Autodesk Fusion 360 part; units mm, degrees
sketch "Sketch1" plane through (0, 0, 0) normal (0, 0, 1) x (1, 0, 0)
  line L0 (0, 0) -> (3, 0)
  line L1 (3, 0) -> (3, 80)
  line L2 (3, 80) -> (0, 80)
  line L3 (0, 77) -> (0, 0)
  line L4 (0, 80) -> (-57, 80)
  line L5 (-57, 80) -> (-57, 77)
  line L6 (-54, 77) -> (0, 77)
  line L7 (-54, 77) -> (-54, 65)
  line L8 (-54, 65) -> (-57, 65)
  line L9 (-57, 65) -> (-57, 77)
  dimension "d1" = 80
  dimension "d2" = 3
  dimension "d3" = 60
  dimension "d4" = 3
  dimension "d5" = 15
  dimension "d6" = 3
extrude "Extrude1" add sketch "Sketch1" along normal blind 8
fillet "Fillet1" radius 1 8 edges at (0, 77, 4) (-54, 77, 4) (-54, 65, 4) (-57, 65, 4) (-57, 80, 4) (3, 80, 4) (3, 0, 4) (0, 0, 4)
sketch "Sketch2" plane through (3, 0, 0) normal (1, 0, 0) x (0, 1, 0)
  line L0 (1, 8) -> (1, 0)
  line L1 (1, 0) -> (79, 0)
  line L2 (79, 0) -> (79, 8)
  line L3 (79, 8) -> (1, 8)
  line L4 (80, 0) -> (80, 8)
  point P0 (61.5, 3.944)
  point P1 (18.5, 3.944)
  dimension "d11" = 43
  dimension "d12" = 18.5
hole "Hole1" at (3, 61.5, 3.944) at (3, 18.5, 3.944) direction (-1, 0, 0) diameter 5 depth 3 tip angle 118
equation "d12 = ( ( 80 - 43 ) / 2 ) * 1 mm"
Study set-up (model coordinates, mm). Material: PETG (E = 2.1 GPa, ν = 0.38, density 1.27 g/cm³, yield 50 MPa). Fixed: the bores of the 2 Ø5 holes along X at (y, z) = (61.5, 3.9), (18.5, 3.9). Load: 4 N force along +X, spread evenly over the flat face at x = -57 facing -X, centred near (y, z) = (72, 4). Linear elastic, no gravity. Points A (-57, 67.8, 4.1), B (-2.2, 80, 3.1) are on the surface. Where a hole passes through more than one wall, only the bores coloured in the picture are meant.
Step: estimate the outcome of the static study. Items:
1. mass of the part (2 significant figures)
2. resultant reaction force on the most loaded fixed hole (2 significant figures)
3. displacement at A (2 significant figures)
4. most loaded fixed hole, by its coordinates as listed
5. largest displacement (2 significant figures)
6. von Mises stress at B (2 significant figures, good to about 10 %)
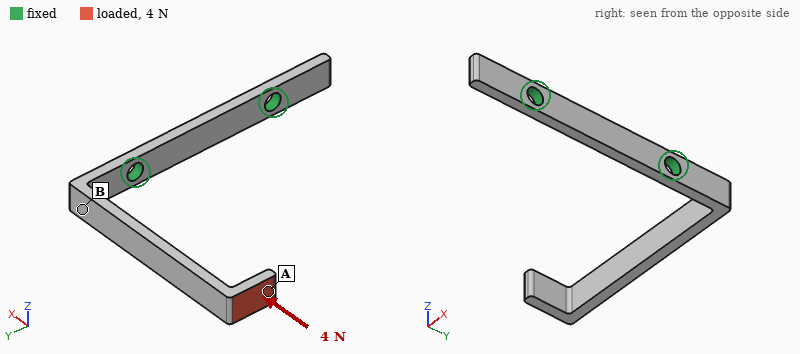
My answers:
4.4 g
4.0 N
0.97 mm
(61.5, 3.9)
1.0 mm
1.7 MPa
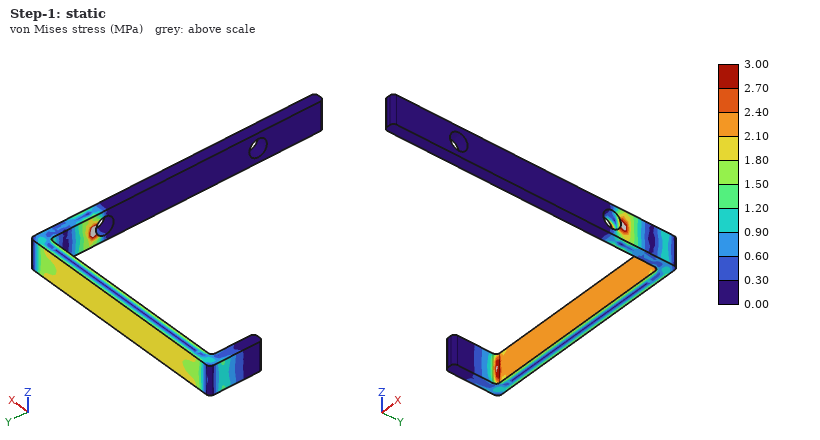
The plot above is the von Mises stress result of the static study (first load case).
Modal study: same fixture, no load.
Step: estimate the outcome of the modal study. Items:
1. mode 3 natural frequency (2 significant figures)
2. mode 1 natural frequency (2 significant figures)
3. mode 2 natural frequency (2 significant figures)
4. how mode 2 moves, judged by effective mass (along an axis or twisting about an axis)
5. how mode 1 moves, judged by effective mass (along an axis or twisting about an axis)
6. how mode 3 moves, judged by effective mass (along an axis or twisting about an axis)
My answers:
570 Hz
100 Hz
150 Hz
along Z
along Y
along X
